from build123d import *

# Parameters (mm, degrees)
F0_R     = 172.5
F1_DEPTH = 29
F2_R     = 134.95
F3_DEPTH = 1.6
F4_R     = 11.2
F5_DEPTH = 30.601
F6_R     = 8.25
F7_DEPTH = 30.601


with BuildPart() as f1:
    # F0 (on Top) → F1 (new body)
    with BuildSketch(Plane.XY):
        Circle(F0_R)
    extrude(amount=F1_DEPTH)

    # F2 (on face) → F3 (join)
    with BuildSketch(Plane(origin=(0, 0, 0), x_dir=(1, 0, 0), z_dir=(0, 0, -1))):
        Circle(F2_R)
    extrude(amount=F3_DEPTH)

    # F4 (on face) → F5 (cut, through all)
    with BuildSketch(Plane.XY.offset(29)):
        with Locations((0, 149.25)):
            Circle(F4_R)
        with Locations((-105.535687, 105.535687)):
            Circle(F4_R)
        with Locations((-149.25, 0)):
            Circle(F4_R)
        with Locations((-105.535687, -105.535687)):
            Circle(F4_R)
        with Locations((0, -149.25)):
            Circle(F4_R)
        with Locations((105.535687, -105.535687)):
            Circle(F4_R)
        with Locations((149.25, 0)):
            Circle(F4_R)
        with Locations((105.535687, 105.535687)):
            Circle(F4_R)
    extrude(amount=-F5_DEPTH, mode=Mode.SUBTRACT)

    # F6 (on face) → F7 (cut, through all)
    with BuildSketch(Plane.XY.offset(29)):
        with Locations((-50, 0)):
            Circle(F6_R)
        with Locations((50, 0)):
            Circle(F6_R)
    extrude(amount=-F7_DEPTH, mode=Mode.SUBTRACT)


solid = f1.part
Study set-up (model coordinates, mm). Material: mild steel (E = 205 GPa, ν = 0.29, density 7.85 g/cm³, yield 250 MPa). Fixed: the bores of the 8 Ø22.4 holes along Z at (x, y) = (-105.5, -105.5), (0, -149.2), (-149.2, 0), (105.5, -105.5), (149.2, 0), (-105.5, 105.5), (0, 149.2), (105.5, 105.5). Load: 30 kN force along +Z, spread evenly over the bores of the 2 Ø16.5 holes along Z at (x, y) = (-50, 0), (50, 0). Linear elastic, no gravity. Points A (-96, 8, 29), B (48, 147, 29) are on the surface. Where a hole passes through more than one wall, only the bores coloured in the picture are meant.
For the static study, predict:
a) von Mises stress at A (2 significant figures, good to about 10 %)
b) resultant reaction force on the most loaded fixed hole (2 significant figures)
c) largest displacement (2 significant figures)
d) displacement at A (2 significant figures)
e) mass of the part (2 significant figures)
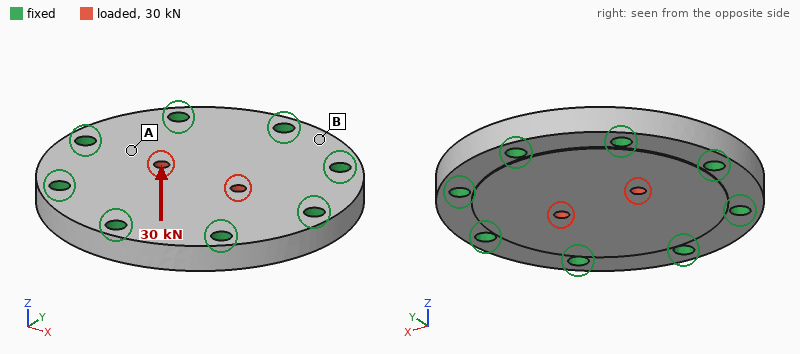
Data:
9.6 MPa
5.2 kN
23 µm
9.4 µm
21 kg
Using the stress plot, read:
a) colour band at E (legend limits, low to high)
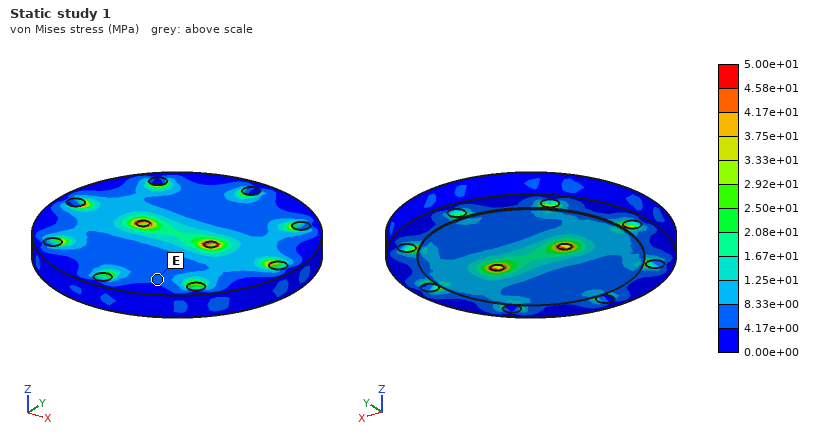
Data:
4.17e+00 to 8.33e+00 MPa
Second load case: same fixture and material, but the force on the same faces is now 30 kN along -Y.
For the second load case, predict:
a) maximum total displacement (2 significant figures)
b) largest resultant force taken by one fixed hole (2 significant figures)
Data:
2.2 µm
5.1 kN
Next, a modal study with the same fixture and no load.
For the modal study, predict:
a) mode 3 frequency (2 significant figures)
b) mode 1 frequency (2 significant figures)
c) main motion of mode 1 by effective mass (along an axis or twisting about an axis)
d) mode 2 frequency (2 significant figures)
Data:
5500 Hz
2800 Hz
along Z
5500 Hz
